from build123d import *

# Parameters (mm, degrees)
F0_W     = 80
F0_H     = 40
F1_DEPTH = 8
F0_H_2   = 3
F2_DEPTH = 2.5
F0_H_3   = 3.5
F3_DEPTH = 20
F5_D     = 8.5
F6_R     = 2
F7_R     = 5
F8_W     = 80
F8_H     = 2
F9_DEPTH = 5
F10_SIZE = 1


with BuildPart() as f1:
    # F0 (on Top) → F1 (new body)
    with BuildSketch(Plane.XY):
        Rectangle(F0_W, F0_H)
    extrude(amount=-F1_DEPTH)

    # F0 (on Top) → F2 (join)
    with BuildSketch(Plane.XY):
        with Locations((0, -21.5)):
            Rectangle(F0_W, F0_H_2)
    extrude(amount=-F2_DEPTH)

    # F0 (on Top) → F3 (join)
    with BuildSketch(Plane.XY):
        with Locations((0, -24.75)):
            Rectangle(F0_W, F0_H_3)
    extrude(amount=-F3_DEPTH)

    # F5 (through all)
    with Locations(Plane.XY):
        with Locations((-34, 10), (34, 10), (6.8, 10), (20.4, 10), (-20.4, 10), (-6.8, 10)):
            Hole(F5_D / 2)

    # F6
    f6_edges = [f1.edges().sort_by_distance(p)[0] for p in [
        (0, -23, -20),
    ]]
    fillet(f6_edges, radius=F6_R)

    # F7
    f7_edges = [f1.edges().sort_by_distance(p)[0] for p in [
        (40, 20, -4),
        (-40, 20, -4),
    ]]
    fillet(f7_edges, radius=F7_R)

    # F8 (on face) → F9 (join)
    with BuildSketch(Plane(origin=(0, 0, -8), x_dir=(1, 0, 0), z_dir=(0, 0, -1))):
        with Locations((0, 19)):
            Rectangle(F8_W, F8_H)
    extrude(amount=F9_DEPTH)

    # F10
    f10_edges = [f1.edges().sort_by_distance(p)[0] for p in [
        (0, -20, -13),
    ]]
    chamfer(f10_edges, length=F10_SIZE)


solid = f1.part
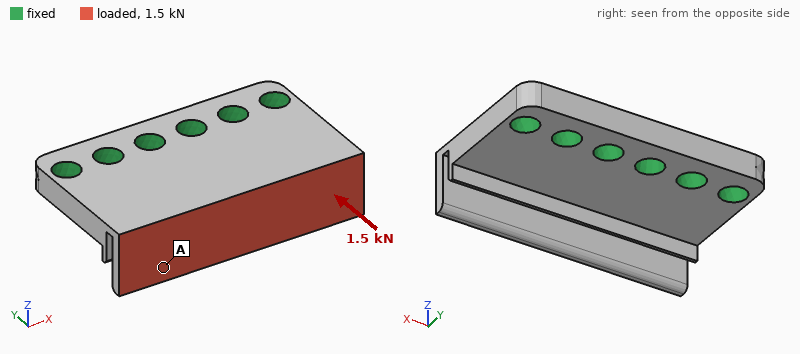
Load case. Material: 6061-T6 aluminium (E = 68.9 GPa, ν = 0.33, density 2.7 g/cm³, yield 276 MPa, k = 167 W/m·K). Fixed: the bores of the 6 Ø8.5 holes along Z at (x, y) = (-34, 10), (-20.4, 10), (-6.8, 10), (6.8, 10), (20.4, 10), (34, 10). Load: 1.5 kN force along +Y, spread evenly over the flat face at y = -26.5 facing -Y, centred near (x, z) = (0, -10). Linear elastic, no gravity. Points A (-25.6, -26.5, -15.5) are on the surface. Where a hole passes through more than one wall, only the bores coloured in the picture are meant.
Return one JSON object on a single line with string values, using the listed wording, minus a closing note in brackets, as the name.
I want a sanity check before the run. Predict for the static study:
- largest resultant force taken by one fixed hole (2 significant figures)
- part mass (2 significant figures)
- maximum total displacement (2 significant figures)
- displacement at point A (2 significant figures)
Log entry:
{"largest resultant force taken by one fixed hole": "280 N", "part mass": "80 g", "maximum total displacement": "0.21 mm", "displacement at point A": "0.16 mm"}
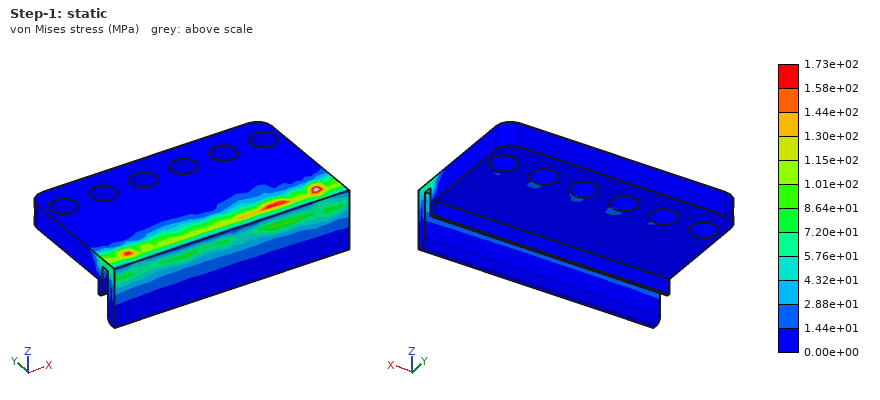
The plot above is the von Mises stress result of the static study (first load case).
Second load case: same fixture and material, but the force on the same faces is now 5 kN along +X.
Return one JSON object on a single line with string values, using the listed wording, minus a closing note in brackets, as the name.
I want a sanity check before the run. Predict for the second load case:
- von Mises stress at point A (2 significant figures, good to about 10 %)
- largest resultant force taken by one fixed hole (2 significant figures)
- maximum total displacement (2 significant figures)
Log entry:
{"von Mises stress at point A": "16 MPa", "largest resultant force taken by one fixed hole": "2.2 kN", "maximum total displacement": "0.11 mm"}
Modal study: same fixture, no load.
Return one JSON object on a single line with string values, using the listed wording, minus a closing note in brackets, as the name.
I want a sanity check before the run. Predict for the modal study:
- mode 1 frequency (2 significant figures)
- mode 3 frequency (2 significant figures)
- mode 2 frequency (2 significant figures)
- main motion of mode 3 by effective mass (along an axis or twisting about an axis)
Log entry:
{"mode 1 frequency": "3800 Hz", "mode 3 frequency": "6000 Hz", "mode 2 frequency": "5000 Hz", "main motion of mode 3 by effective mass": "along Z"}
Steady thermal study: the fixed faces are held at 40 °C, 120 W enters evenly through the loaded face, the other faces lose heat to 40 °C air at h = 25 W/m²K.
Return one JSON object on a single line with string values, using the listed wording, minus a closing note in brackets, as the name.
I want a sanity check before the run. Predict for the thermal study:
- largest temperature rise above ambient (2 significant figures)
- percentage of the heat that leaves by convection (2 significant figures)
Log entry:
{"largest temperature rise above ambient": "68 K", "percentage of the heat that leaves by convection": "5.0 %"}
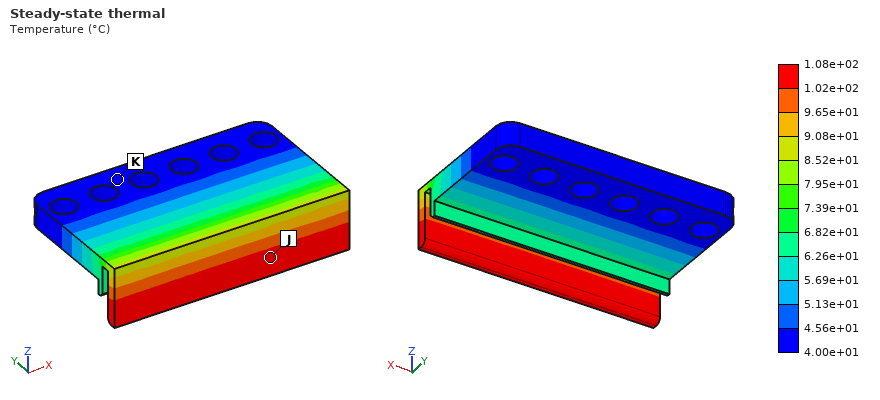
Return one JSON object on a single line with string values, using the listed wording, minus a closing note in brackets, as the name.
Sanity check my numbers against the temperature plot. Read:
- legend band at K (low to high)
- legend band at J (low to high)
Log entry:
{"legend band at K": "4.00e+01 to 4.56e+01 °C", "legend band at J": "1.02e+02 to 1.08e+02 °C"}
